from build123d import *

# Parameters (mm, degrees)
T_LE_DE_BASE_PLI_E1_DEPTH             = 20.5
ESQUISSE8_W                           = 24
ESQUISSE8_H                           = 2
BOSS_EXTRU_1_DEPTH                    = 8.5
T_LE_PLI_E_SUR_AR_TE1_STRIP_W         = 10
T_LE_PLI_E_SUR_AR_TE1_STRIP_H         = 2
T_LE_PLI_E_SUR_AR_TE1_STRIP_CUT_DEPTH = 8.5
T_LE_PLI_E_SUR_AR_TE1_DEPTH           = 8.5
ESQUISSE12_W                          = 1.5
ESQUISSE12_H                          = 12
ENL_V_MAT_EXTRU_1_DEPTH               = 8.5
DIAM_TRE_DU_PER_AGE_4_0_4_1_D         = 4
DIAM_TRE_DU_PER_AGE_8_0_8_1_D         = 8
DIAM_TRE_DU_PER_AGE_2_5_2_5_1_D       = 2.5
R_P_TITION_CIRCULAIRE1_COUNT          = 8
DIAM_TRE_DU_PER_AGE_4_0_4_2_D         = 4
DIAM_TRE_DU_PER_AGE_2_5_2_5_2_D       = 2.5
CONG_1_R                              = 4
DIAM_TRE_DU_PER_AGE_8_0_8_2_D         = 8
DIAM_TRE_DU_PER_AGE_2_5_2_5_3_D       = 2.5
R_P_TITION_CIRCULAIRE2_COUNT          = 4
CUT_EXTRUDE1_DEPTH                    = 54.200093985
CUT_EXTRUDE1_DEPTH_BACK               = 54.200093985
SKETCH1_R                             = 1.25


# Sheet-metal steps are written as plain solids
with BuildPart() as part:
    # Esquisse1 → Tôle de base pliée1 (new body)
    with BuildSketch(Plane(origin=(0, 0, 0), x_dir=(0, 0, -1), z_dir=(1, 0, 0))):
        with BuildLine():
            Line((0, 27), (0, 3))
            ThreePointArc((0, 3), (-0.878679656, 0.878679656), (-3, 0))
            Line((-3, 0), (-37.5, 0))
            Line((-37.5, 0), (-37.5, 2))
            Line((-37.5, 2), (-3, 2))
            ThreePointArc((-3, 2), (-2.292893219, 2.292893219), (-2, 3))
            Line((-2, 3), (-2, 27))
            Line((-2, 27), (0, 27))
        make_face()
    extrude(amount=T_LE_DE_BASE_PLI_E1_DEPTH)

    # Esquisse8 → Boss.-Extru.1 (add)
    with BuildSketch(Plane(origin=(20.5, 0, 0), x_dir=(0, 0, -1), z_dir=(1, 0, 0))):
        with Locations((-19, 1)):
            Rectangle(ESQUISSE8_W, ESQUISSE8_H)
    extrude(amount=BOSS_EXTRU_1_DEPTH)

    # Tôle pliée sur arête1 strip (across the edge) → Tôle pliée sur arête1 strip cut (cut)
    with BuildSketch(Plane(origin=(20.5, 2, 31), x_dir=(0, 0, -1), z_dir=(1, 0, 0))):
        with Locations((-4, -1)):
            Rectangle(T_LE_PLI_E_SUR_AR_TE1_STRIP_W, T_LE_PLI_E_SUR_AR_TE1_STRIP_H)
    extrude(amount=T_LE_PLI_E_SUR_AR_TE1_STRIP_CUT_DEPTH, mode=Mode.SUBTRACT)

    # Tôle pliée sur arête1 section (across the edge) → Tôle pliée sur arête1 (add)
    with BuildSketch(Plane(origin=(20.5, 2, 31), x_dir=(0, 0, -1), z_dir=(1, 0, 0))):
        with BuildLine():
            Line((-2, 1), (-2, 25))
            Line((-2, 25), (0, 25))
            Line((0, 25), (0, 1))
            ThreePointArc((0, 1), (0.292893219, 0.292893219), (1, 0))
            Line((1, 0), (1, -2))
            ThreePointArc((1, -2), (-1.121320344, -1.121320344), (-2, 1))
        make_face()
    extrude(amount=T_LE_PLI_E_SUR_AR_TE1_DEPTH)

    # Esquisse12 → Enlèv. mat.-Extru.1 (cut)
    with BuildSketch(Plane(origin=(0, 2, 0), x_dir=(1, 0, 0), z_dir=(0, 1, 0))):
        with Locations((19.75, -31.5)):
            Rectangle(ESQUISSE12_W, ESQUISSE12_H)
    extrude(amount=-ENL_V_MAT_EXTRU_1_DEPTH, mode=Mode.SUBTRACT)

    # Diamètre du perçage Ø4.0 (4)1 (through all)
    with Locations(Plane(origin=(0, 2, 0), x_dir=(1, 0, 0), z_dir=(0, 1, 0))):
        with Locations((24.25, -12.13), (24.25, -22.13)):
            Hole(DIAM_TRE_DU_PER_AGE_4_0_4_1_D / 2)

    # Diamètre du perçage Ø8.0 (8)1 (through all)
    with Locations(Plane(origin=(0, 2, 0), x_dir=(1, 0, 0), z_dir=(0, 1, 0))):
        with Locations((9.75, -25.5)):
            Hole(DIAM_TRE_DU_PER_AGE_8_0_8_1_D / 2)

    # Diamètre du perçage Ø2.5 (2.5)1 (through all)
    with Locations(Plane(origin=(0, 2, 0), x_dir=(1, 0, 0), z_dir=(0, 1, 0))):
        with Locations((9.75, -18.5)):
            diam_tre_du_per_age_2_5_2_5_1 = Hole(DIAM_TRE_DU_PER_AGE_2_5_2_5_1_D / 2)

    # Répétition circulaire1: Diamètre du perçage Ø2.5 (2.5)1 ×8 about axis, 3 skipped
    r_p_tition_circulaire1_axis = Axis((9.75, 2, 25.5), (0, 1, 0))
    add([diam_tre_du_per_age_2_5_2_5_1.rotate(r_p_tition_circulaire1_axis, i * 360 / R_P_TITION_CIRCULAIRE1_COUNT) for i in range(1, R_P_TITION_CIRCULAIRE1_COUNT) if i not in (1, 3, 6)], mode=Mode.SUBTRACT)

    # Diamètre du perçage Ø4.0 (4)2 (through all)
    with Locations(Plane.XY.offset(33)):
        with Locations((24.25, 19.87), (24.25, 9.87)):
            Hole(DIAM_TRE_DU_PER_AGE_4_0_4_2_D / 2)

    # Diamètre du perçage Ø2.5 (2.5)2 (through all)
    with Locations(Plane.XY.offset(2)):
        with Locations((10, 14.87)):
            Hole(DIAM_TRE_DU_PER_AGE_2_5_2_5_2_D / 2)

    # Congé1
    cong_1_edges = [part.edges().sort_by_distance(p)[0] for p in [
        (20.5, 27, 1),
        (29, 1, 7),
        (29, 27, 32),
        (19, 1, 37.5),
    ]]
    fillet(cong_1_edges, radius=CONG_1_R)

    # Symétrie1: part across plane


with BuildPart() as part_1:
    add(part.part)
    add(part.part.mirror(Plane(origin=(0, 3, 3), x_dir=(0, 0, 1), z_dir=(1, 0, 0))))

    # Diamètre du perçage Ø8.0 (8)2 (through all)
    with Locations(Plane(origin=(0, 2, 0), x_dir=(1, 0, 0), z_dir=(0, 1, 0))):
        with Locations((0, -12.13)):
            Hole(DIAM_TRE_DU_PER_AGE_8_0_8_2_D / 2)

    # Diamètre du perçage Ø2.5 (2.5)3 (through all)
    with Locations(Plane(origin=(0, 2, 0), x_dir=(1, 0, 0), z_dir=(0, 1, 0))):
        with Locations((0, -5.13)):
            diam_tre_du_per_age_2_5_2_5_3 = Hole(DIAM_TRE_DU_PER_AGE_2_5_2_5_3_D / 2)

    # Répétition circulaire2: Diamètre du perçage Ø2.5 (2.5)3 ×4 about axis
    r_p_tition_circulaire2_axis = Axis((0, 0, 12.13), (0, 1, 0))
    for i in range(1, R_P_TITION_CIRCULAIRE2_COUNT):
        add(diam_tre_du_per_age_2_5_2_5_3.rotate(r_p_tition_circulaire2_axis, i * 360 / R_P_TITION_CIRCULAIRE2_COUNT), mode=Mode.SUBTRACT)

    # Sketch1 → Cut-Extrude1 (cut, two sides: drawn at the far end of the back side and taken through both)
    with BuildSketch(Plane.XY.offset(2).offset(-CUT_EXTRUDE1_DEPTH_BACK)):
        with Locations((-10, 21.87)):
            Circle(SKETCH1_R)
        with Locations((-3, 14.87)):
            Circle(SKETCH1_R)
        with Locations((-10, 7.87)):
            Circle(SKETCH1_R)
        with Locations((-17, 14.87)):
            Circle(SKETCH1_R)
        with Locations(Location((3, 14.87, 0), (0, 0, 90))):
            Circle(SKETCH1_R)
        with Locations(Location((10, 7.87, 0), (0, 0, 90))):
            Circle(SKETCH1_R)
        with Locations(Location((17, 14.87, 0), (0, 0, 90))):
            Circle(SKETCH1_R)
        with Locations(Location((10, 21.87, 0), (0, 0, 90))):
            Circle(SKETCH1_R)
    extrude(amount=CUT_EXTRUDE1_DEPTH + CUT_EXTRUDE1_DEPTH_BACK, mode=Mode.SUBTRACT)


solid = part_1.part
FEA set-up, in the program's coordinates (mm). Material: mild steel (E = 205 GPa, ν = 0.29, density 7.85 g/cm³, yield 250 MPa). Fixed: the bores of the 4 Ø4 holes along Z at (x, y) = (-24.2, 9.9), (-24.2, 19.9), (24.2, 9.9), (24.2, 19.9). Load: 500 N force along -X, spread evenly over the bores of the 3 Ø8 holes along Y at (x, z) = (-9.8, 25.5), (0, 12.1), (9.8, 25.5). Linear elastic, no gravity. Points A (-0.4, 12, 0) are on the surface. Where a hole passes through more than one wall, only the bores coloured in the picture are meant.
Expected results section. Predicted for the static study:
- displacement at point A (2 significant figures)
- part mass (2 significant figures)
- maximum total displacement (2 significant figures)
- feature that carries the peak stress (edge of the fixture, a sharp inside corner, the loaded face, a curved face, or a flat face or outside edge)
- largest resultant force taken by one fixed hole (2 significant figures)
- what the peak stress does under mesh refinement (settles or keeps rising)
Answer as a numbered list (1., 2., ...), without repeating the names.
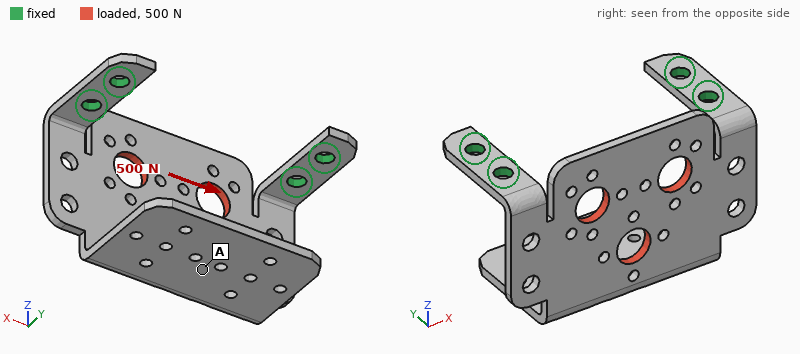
1. 33 µm
2. 46 g
3. 47 µm
4. edge of the fixture
5. 310 N
6. keeps rising
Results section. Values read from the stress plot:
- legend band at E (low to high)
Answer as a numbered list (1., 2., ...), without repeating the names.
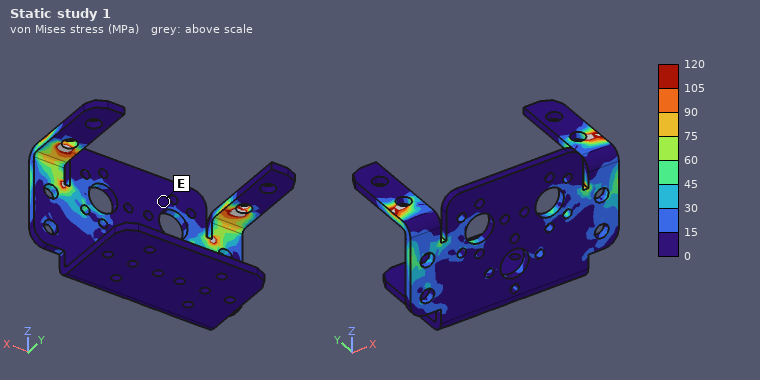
1. 0 to 15 MPa
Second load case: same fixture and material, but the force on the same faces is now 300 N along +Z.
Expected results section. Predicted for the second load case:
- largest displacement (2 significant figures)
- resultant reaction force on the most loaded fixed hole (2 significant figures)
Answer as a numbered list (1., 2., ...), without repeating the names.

1. 0.13 mm
2. 160 N
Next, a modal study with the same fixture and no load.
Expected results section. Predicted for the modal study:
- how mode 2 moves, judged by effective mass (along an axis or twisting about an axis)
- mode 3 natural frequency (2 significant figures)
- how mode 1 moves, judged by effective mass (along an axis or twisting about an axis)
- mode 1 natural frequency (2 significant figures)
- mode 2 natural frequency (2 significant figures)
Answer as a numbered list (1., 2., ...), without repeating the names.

1. along X
2. 1500 Hz
3. along Y
4. 380 Hz
5. 1100 Hz
